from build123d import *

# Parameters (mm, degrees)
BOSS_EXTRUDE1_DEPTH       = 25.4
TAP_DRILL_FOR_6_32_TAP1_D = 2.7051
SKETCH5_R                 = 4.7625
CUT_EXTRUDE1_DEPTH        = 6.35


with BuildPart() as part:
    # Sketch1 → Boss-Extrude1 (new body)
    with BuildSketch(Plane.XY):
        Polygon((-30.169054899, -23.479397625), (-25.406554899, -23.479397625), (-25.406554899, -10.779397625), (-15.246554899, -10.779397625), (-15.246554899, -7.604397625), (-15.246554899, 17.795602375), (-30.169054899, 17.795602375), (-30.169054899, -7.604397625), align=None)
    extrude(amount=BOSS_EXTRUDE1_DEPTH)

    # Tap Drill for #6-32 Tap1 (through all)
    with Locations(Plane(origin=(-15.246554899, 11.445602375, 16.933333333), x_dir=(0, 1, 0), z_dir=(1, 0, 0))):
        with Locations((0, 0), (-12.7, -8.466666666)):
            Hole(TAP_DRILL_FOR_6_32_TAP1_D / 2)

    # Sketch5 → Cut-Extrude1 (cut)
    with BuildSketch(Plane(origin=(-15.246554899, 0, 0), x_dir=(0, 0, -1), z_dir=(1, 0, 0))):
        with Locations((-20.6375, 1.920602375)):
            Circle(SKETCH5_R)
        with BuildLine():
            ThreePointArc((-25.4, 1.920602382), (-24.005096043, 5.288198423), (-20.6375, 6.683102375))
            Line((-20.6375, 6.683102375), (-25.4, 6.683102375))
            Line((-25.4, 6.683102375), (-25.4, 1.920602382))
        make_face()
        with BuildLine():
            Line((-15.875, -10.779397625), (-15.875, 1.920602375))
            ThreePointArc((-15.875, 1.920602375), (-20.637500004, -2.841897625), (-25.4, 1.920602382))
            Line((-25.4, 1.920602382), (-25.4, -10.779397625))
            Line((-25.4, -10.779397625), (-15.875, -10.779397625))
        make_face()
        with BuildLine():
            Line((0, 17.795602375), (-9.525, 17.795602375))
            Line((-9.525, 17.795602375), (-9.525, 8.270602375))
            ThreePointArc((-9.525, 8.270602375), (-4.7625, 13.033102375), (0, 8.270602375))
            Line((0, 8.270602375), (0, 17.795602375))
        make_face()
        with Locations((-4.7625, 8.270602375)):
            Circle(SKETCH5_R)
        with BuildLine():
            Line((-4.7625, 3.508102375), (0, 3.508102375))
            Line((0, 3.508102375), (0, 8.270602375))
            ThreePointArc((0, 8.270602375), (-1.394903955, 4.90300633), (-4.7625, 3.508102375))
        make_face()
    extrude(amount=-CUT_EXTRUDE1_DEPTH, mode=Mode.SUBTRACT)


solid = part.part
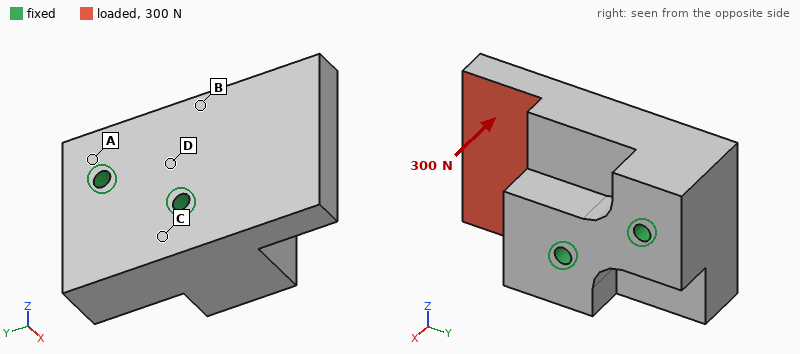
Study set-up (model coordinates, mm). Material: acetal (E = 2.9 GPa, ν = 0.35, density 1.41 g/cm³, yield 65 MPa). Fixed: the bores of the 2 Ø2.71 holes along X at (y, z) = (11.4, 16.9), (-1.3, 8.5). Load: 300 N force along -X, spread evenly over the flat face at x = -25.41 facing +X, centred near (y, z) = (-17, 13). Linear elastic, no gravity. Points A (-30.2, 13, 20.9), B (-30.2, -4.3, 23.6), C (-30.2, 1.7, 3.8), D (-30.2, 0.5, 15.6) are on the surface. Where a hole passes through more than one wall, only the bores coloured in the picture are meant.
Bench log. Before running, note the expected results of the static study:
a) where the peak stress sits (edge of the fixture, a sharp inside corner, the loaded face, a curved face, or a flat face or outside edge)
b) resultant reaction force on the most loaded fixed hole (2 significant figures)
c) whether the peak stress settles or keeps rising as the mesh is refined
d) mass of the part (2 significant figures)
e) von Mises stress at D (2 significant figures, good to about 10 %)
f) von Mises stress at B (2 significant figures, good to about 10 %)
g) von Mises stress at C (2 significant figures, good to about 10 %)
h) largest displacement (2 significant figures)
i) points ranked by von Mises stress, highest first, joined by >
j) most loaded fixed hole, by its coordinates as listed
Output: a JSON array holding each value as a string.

["edge of the fixture", "350 N", "keeps rising", "15 g", "4.7 MPa", "6.6 MPa", "3.0 MPa", "0.36 mm", "B > D > C > A", "(-1.3, 8.5)"]
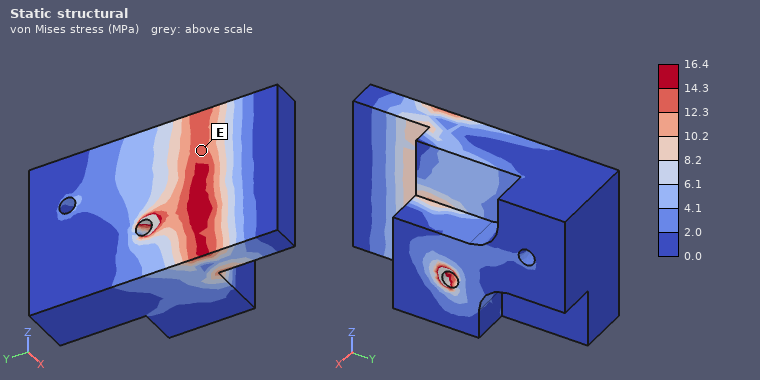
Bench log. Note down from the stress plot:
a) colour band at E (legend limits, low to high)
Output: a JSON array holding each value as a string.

["12.3 to 14.3 MPa"]
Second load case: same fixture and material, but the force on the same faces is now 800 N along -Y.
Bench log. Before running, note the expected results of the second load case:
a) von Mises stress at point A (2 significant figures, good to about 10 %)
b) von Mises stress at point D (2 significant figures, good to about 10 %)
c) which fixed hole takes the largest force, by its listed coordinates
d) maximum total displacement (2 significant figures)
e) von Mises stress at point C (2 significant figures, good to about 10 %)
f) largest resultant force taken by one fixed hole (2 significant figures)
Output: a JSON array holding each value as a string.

["1.8 MPa", "3.0 MPa", "(-1.3, 8.5)", "0.23 mm", "2.0 MPa", "500 N"]
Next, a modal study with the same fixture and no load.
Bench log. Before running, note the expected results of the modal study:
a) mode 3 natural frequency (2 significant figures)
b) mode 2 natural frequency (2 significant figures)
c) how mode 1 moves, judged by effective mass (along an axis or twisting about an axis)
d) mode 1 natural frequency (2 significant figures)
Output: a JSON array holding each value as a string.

["6000 Hz", "5900 Hz", "along X", "3900 Hz"]
